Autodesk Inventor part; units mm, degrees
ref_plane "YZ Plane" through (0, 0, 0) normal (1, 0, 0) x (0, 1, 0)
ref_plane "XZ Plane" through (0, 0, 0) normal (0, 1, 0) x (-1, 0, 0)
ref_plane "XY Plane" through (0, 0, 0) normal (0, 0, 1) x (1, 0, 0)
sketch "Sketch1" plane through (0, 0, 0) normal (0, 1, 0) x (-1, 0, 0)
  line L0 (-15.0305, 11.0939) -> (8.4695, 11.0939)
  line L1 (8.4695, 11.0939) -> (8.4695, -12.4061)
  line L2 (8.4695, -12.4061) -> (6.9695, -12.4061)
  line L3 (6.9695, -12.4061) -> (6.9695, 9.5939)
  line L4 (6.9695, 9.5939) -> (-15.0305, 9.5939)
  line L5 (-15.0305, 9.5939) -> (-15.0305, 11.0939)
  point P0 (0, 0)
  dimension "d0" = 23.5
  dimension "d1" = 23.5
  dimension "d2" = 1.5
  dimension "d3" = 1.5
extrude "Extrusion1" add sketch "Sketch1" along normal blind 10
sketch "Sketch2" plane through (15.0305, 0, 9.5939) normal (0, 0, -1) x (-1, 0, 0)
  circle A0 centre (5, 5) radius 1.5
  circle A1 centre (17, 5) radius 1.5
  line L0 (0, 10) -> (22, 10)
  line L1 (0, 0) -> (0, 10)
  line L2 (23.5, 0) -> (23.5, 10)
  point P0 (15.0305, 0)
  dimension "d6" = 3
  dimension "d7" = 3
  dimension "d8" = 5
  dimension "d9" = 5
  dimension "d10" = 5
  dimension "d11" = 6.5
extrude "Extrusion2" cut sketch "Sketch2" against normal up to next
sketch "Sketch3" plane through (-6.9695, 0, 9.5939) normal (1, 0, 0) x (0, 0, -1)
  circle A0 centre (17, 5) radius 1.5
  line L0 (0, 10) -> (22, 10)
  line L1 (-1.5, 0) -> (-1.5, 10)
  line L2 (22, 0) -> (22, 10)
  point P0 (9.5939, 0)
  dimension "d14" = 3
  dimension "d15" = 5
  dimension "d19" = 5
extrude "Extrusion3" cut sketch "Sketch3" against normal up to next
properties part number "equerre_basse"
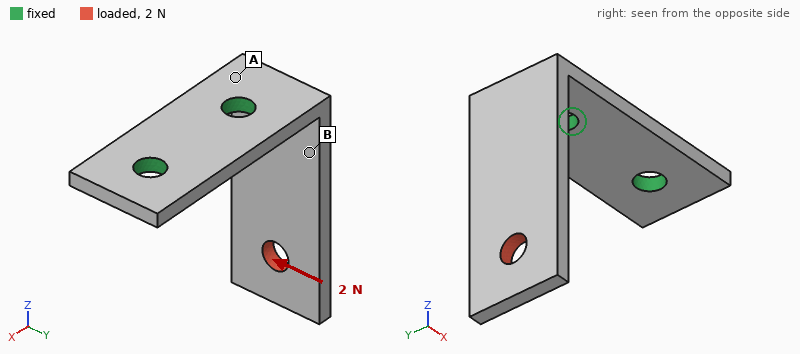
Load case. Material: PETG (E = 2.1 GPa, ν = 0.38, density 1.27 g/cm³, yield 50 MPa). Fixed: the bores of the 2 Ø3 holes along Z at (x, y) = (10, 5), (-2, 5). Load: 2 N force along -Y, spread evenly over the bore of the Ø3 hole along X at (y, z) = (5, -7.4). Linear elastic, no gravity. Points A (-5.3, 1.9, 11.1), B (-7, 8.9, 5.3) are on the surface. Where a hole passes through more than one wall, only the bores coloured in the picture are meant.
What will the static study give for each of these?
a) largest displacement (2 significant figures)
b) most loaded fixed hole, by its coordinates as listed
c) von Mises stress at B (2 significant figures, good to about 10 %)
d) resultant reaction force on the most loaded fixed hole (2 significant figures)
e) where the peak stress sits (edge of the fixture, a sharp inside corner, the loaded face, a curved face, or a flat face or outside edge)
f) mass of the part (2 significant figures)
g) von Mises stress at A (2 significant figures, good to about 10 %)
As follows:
0.36 mm
(-2, 5)
1.6 MPa
2.5 N
a flat face or outside edge
0.83 g
3.8 MPa
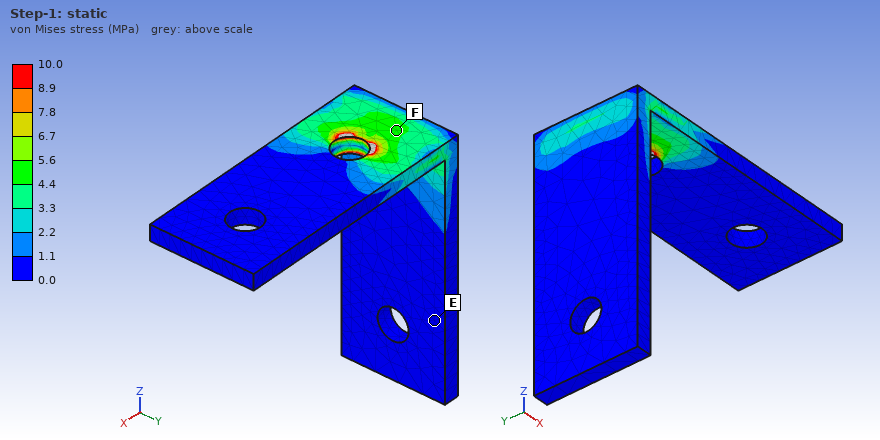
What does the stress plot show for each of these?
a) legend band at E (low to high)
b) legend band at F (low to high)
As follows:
0.0 to 1.1 MPa
4.4 to 5.6 MPa
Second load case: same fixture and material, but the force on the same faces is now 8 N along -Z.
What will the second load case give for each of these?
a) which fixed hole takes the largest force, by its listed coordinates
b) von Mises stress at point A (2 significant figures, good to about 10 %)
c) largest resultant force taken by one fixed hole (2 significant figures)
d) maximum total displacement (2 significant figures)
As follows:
(-2, 5)
4.2 MPa
8.2 N
0.37 mm
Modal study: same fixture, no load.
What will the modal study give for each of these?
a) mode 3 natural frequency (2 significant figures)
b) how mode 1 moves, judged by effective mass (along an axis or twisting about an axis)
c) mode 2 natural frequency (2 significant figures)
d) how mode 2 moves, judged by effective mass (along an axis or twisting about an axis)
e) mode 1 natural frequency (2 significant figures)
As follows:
2600 Hz
along X
890 Hz
along Y
480 Hz
